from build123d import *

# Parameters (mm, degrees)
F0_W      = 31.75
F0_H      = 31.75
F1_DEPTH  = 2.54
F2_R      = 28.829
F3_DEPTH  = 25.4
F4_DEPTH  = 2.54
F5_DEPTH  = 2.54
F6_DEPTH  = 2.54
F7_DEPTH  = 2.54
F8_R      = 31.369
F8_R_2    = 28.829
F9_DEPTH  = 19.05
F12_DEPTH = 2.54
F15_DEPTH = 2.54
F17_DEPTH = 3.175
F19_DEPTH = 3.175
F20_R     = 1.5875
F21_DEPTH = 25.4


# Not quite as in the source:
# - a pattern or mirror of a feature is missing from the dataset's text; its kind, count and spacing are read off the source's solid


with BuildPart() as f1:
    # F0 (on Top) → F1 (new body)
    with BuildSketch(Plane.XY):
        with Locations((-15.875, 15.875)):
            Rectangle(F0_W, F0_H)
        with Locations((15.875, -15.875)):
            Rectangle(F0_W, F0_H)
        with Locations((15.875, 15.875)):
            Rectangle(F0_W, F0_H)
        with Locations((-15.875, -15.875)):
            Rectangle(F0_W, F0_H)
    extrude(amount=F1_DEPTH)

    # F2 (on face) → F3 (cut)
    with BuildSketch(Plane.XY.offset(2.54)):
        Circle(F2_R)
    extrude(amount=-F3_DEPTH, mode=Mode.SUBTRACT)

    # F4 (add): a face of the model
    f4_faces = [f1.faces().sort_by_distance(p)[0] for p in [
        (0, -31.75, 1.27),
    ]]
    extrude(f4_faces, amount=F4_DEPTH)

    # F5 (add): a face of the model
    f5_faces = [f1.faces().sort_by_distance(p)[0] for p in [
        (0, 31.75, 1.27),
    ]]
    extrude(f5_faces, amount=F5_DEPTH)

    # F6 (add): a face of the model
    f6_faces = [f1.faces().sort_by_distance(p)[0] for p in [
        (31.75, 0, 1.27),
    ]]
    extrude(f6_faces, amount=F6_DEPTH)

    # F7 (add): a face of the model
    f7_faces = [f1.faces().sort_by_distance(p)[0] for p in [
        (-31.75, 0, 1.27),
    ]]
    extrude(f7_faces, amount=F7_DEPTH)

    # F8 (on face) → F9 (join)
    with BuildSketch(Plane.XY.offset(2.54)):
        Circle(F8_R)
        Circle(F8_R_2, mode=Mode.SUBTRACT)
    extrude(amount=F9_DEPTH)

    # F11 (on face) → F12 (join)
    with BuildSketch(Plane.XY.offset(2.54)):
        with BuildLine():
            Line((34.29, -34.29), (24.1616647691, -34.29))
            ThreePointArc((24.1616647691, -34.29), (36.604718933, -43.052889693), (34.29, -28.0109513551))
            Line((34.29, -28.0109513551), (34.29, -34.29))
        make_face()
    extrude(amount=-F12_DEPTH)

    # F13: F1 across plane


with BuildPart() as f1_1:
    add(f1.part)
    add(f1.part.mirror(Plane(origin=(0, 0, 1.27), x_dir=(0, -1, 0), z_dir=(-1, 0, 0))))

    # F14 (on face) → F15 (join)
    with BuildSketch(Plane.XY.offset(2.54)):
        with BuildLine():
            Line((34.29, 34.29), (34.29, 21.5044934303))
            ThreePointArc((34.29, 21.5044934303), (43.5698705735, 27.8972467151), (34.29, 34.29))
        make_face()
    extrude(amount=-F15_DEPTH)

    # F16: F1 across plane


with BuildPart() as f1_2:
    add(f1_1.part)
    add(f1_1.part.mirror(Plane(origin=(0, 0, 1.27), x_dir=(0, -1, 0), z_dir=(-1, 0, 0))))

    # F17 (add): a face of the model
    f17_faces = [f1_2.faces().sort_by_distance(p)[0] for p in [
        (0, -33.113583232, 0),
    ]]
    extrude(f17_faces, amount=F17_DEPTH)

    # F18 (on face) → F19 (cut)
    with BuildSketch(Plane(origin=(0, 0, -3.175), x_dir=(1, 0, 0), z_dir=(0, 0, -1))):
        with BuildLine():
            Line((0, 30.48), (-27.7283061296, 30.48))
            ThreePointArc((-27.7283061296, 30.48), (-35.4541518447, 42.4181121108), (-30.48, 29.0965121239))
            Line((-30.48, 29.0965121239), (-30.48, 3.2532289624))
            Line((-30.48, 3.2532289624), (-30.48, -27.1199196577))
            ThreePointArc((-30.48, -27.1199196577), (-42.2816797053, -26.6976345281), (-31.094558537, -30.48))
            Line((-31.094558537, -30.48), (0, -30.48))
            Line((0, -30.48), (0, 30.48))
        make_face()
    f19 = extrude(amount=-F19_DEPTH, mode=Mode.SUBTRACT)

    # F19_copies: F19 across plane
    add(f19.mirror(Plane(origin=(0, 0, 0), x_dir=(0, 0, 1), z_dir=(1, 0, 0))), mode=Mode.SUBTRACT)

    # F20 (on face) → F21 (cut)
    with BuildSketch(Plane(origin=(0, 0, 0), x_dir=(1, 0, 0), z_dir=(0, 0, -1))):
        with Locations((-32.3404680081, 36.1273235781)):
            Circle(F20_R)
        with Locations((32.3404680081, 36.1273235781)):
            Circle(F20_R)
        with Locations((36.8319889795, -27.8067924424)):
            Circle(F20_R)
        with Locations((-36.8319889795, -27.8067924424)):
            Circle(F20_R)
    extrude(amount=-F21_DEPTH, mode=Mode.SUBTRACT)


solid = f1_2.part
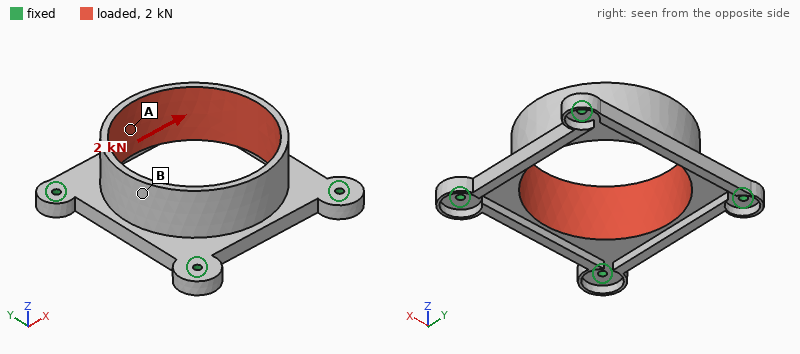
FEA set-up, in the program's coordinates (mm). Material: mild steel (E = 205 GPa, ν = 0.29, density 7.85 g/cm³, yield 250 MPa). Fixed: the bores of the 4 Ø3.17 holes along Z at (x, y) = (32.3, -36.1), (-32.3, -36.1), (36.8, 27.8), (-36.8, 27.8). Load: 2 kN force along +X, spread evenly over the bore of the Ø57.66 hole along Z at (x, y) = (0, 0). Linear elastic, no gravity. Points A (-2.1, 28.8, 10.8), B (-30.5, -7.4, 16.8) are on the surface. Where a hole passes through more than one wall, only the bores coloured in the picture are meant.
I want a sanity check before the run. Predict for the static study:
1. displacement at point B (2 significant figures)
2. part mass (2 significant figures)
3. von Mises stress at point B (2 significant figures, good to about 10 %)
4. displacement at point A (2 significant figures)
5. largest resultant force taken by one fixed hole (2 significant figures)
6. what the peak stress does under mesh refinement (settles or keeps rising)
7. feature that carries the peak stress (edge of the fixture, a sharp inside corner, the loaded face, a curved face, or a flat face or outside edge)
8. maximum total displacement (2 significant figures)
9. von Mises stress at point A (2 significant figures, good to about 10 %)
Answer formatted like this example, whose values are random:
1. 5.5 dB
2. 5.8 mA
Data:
1. 19 µm
2. 150 g
3. 15 MPa
4. 5.2 µm
5. 570 N
6. keeps rising
7. edge of the fixture
8. 22 µm
9. 7.3 MPa
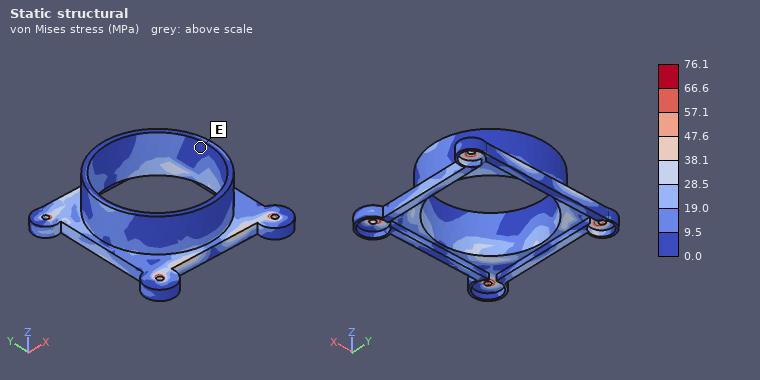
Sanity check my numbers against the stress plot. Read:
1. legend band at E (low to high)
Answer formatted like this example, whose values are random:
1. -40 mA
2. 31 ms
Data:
1. 0.0 to 9.5 MPa
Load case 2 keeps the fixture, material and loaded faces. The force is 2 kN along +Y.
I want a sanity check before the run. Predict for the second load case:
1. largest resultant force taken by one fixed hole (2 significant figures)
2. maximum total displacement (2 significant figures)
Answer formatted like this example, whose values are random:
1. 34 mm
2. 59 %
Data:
1. 640 N
2. 30 µm
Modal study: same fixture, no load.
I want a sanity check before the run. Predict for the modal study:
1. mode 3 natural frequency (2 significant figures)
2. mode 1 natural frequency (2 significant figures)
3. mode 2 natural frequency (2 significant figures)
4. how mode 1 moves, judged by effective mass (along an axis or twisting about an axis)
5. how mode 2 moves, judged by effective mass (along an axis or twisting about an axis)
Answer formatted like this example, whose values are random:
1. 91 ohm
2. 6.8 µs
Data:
1. 4100 Hz
2. 3500 Hz
3. 3800 Hz
4. along Z
5. along Z
